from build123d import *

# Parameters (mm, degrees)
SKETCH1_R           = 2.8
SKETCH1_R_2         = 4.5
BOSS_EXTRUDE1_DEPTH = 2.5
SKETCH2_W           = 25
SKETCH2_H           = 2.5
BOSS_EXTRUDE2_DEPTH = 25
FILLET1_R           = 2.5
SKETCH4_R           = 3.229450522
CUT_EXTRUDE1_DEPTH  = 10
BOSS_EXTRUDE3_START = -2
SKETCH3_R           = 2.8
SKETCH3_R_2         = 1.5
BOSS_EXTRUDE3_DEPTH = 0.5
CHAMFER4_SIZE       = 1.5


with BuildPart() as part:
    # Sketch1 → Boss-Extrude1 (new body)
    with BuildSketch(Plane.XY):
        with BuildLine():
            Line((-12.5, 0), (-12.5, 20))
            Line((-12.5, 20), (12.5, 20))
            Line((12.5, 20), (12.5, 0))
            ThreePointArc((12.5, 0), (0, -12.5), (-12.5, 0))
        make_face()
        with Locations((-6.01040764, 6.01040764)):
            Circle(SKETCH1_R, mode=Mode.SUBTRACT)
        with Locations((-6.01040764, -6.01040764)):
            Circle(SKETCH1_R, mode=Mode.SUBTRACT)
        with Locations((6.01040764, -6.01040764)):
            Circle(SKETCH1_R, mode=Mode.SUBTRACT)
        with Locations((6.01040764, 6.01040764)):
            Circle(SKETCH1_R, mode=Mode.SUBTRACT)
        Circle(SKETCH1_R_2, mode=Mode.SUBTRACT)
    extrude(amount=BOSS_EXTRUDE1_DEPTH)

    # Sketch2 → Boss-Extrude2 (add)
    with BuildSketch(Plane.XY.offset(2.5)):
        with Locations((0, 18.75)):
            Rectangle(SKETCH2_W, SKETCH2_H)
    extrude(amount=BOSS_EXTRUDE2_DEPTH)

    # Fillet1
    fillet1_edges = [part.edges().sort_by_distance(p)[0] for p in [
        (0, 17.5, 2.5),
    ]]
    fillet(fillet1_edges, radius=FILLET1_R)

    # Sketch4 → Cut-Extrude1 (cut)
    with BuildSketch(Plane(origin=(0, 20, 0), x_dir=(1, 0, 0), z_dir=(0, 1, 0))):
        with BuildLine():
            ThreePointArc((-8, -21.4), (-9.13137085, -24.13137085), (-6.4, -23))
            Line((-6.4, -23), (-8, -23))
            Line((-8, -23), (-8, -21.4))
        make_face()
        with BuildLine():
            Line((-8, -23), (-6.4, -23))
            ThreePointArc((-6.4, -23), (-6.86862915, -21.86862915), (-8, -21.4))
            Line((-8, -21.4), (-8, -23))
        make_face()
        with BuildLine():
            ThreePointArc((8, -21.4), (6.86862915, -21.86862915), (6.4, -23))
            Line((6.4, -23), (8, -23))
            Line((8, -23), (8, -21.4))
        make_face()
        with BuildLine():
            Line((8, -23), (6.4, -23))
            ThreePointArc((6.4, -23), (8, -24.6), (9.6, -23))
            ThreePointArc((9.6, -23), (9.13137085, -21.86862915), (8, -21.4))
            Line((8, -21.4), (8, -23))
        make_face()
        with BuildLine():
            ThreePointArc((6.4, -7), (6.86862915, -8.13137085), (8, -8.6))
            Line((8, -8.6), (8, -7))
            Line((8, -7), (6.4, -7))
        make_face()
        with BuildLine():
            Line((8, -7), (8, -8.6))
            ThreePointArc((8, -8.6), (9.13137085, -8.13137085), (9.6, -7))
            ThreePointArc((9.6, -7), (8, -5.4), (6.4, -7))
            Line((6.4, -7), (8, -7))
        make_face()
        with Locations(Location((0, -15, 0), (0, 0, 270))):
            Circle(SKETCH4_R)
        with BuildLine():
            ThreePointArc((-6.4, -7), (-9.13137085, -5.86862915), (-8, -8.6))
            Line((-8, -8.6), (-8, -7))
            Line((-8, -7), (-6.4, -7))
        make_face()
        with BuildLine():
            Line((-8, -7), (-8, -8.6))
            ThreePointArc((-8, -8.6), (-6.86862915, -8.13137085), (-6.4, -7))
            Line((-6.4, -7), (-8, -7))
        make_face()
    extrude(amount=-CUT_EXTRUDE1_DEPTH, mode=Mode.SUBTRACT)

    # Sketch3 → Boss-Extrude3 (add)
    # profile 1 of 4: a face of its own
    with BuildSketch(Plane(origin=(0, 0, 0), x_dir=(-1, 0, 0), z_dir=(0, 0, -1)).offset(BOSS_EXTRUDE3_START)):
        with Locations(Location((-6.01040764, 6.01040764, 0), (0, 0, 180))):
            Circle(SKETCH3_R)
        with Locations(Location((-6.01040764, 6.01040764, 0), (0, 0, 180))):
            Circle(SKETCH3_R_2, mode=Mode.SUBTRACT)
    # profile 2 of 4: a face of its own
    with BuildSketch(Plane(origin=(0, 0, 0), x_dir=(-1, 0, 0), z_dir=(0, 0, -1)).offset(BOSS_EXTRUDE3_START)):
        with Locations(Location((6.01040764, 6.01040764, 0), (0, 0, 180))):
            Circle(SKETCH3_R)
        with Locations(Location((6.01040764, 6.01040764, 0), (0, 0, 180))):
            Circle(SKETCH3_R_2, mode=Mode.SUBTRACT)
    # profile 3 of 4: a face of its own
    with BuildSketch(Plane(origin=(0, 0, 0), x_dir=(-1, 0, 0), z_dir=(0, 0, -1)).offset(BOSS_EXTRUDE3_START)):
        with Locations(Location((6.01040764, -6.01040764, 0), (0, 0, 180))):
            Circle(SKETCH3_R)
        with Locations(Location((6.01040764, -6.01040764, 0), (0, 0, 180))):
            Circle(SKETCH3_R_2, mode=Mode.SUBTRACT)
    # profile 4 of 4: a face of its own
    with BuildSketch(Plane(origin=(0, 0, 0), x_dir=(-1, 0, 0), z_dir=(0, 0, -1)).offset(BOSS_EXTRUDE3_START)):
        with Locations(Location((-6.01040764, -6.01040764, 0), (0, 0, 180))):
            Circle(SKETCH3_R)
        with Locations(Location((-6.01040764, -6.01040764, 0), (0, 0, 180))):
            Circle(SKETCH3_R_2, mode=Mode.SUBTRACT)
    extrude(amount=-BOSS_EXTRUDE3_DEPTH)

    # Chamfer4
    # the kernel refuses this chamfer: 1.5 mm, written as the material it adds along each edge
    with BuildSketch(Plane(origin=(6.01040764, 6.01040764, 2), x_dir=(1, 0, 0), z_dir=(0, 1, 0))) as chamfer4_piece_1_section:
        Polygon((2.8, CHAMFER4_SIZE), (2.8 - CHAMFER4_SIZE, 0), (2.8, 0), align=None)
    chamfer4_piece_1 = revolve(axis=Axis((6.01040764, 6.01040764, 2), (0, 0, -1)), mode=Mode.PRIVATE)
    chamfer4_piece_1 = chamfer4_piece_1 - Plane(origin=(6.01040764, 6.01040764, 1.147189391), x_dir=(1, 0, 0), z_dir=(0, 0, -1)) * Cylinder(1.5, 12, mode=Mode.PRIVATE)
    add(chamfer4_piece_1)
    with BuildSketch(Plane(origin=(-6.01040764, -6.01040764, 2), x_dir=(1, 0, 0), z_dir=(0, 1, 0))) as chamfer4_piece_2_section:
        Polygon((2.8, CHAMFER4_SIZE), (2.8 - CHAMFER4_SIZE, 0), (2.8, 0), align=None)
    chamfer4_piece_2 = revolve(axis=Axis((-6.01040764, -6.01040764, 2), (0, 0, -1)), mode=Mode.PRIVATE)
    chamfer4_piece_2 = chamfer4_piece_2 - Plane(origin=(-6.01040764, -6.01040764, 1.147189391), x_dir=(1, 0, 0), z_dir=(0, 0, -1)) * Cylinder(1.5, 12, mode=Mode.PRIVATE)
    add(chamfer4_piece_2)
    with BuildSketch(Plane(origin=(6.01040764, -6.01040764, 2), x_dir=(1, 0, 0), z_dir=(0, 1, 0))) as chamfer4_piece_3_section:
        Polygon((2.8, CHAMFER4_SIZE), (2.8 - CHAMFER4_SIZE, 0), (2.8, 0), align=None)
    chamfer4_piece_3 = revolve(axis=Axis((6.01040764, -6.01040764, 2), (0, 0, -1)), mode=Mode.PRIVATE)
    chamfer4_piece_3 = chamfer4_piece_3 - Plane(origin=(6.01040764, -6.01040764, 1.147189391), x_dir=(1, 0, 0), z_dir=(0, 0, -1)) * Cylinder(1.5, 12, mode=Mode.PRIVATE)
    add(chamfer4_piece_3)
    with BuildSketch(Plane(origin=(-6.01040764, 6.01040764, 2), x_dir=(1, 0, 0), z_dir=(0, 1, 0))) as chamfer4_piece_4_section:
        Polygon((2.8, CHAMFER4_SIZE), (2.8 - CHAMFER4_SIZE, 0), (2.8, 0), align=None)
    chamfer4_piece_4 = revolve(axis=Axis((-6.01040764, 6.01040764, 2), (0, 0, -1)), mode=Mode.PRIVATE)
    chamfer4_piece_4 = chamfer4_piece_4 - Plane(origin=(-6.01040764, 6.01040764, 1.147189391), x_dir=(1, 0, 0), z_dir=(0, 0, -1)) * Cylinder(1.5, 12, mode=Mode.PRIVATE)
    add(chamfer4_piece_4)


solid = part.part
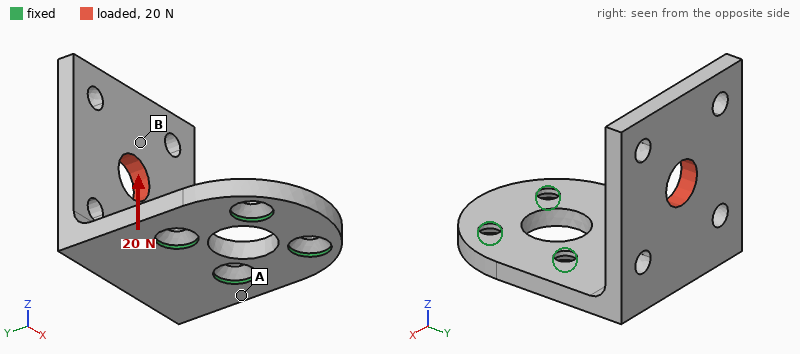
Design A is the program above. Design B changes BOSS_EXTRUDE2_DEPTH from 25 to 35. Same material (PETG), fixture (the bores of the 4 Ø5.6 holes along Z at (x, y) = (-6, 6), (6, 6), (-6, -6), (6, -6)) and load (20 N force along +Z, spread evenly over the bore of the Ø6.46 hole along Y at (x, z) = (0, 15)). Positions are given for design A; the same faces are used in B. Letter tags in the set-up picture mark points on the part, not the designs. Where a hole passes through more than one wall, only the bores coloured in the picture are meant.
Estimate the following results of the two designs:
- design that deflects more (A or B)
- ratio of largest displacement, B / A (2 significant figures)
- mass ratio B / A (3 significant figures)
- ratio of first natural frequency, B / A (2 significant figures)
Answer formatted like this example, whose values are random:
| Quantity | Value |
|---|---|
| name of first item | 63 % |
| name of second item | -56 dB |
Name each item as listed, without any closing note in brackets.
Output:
| Quantity | Value |
|---|---|
| design that deflects more | B |
| ratio of largest displacement, B / A | 1.3 |
| mass ratio B / A | 1.21 |
| ratio of first natural frequency, B / A | 0.57 |
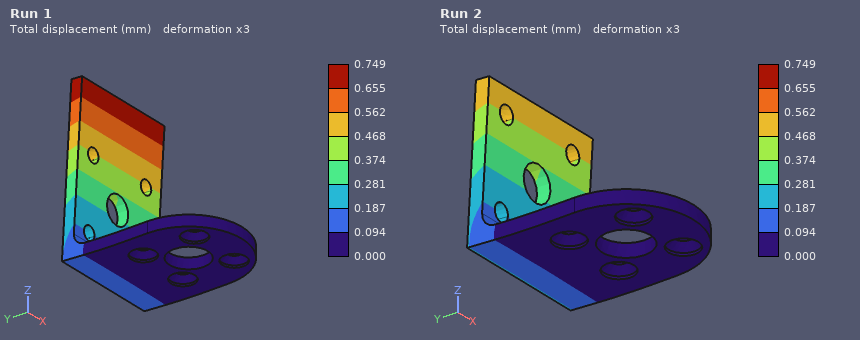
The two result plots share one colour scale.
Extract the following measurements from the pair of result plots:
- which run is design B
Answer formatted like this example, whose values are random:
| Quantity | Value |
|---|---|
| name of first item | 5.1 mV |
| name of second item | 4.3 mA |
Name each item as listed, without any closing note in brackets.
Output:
| Quantity | Value |
|---|---|
| which run is design B | Run 1 |
